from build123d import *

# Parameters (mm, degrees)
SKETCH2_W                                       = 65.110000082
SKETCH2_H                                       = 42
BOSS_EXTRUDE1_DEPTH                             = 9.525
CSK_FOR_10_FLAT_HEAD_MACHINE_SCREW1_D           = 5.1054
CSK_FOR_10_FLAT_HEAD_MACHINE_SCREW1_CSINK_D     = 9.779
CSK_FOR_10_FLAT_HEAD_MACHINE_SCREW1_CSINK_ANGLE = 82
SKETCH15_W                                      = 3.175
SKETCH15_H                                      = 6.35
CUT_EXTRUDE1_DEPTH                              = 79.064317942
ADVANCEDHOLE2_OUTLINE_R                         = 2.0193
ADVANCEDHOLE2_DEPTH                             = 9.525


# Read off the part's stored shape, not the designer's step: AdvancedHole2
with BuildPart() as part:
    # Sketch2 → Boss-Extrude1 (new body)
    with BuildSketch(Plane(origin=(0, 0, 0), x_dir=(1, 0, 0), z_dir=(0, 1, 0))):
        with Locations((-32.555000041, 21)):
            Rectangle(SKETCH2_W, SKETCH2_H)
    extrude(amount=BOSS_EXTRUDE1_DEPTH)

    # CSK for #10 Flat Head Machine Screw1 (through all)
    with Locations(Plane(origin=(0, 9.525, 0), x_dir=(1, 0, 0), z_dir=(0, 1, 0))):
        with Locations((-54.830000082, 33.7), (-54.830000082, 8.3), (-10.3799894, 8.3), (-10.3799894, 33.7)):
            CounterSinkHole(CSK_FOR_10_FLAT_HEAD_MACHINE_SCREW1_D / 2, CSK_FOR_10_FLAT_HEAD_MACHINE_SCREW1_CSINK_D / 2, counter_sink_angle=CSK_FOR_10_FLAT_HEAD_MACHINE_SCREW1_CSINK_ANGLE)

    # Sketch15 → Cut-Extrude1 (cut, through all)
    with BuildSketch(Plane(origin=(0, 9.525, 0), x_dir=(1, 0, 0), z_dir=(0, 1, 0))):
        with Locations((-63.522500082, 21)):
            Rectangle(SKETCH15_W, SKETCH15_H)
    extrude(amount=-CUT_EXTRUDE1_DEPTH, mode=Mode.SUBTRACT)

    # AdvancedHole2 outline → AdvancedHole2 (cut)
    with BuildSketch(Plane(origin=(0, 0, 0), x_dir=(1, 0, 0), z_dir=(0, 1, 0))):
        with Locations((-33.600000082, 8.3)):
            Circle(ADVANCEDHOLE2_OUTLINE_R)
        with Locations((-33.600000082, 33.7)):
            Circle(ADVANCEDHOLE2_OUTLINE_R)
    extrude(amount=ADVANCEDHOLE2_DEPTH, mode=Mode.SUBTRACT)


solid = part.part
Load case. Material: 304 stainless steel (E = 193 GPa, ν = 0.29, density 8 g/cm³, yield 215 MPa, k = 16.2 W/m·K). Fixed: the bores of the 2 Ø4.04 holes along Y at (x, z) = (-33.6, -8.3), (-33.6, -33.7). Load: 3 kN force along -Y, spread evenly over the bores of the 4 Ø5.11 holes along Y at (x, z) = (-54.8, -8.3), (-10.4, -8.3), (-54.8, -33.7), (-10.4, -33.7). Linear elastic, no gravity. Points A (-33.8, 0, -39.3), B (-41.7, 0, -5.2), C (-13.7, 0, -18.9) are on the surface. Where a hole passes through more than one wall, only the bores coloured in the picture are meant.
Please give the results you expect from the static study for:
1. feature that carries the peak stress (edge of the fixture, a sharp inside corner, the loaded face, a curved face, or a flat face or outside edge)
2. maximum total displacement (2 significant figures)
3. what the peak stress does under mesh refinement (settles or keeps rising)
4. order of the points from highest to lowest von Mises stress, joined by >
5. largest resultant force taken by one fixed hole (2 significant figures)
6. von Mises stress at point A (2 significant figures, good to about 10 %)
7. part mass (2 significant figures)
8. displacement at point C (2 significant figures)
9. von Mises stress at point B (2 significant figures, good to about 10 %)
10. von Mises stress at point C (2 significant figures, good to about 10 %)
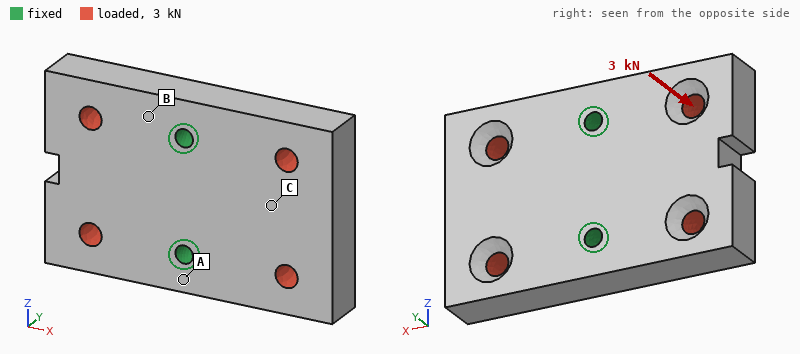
edge of the fixture
19 µm
keeps rising
A > B > C
1.5 kN
44 MPa
200 g
9.5 µm
30 MPa
9.1 MPa
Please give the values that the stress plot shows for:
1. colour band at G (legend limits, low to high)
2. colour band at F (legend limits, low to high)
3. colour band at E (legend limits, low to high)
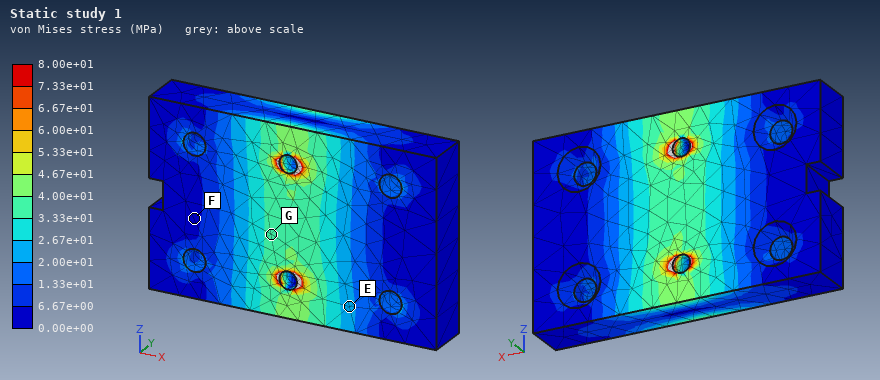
3.33e+01 to 4.00e+01 MPa
0.00e+00 to 6.67e+00 MPa
2.00e+01 to 2.67e+01 MPa
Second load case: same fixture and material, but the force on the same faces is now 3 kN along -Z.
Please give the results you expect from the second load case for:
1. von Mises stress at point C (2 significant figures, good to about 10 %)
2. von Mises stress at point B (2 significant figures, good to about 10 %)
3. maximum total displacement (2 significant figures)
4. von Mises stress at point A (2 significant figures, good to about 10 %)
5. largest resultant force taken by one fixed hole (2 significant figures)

9.4 MPa
7.6 MPa
2.9 µm
10.0 MPa
1.5 kN
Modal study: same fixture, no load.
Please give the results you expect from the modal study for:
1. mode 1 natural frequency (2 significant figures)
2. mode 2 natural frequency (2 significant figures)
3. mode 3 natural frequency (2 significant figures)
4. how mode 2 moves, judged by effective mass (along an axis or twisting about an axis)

5600 Hz
7400 Hz
12 kHz
along Y
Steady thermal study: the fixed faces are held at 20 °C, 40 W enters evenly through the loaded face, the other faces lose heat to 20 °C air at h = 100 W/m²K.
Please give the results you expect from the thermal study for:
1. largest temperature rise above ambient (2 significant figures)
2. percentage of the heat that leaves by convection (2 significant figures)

56 K
54 %
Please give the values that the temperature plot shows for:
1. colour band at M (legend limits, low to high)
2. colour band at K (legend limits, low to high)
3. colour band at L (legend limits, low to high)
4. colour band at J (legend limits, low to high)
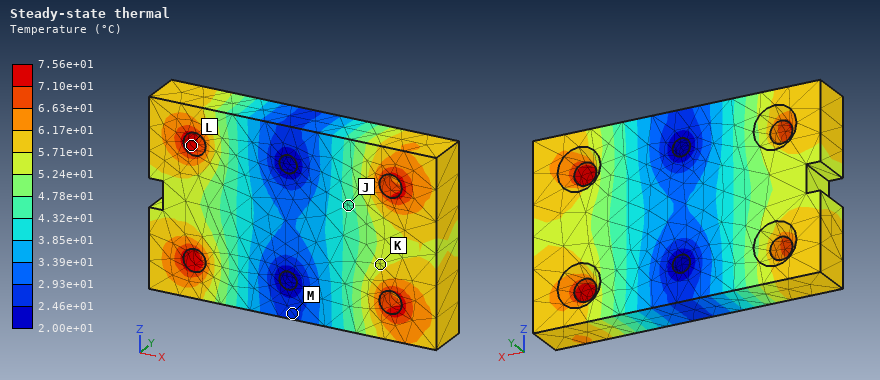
2.46e+01 to 2.93e+01 °C
5.24e+01 to 5.71e+01 °C
7.10e+01 to 7.56e+01 °C
4.32e+01 to 4.78e+01 °C
